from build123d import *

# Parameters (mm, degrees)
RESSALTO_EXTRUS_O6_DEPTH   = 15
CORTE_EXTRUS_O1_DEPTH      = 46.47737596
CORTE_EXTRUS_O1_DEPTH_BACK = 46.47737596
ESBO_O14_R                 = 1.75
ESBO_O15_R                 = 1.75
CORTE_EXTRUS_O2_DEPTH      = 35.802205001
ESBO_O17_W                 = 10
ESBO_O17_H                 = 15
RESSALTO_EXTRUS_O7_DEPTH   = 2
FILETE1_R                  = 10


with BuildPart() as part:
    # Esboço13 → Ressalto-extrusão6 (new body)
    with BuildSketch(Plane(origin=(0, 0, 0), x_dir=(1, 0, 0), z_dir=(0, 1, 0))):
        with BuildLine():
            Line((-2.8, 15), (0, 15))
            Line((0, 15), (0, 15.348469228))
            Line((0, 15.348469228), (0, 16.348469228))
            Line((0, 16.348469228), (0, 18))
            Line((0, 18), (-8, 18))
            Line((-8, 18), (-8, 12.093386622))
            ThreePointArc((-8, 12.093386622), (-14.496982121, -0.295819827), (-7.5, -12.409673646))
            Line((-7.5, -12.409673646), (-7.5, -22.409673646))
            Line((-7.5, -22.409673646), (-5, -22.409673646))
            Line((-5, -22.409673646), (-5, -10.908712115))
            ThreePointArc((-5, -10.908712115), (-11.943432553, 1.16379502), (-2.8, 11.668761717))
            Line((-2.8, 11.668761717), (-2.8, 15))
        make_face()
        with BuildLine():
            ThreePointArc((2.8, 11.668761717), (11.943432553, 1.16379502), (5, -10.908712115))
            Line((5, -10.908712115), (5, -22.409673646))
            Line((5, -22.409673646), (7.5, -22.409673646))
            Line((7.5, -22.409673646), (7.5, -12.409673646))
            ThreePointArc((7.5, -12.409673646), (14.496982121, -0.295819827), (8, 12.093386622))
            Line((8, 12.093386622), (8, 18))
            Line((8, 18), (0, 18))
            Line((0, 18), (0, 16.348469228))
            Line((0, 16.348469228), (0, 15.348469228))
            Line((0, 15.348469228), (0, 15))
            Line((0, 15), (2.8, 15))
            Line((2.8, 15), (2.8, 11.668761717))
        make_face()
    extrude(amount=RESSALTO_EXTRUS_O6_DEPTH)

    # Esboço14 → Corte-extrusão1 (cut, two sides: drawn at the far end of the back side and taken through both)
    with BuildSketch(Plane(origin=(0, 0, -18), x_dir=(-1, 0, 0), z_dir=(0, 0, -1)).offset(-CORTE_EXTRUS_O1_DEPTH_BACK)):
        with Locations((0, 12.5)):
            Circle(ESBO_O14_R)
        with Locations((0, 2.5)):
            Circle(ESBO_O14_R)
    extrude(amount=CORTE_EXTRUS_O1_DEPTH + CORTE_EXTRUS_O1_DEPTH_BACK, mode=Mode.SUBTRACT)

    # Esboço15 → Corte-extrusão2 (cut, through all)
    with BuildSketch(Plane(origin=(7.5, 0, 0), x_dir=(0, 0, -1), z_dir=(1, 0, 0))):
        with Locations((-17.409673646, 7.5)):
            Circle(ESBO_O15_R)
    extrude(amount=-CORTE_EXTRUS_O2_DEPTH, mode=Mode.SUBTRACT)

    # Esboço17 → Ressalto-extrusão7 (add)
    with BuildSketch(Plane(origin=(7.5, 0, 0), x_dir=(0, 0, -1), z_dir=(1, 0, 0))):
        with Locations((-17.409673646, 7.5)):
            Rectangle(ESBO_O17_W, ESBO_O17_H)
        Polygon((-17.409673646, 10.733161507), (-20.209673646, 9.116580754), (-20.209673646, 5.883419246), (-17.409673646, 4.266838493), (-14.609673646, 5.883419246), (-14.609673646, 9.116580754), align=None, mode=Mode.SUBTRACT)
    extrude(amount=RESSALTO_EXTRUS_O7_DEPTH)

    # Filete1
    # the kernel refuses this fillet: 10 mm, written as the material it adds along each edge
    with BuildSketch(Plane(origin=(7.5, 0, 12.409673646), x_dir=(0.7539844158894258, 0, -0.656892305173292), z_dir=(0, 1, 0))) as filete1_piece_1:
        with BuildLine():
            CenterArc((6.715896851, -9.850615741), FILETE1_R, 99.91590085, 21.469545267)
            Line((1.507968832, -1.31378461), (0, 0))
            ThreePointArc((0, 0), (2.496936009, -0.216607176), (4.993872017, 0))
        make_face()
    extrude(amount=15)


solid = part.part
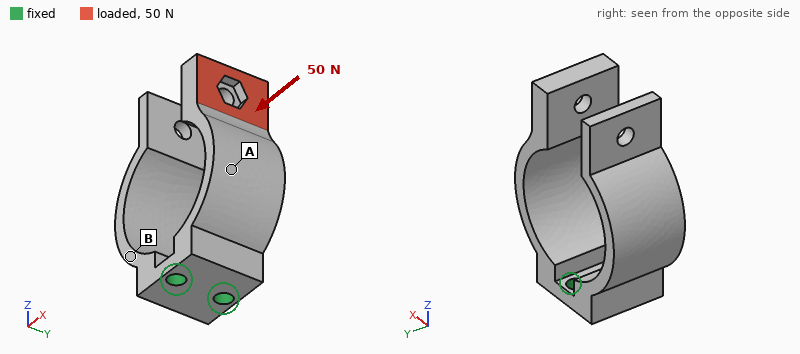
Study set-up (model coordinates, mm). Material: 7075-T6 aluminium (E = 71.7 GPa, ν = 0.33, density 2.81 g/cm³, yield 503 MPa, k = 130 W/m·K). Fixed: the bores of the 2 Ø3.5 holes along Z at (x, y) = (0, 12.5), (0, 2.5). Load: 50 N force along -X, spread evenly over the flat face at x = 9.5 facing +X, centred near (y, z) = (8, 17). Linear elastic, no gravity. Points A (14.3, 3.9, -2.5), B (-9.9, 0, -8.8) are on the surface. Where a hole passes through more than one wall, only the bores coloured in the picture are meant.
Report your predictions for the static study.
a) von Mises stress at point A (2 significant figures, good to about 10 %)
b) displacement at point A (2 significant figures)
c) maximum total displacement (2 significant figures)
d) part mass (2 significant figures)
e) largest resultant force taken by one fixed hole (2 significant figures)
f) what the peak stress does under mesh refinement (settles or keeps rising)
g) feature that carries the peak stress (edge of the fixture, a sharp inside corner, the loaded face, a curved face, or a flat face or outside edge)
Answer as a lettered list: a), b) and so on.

a) 54 MPa
b) 0.11 mm
c) 0.53 mm
d) 12 g
e) 32 N
f) keeps rising
g) edge of the fixture
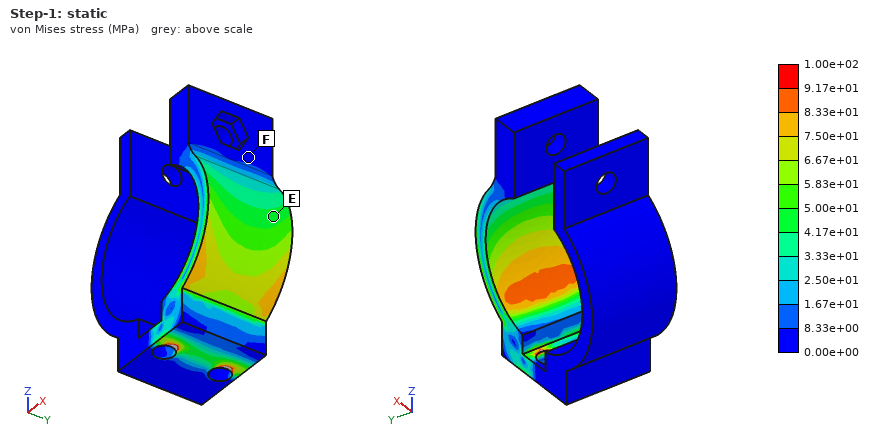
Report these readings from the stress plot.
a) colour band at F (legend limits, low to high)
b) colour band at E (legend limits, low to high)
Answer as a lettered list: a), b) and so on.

a) 0.00e+00 to 8.33e+00 MPa
b) 4.17e+01 to 5.00e+01 MPa
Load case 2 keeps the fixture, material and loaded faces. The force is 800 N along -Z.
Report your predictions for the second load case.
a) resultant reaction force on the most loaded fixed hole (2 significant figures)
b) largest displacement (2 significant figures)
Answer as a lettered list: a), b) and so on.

a) 400 N
b) 0.28 mm
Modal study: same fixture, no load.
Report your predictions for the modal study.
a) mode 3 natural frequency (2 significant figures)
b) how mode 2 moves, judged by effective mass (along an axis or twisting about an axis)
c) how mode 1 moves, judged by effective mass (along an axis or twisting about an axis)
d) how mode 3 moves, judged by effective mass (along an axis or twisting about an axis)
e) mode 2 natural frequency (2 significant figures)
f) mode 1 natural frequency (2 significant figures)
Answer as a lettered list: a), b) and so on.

a) 2300 Hz
b) along X
c) along X
d) along Y
e) 1400 Hz
f) 1100 Hz
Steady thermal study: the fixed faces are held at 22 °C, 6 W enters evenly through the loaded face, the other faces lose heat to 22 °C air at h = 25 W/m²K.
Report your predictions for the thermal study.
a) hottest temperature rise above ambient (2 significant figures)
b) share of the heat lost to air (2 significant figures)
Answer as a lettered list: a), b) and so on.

a) 39 K
b) 15 %
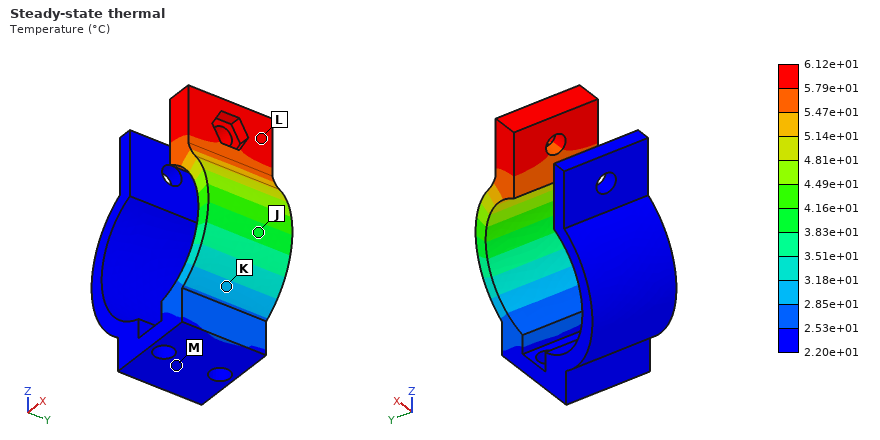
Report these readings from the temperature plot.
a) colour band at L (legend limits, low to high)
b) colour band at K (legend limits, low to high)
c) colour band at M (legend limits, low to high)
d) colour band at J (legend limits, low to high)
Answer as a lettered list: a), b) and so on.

a) 5.79e+01 to 6.12e+01 °C
b) 2.85e+01 to 3.18e+01 °C
c) 2.20e+01 to 2.53e+01 °C
d) 3.83e+01 to 4.16e+01 °C
